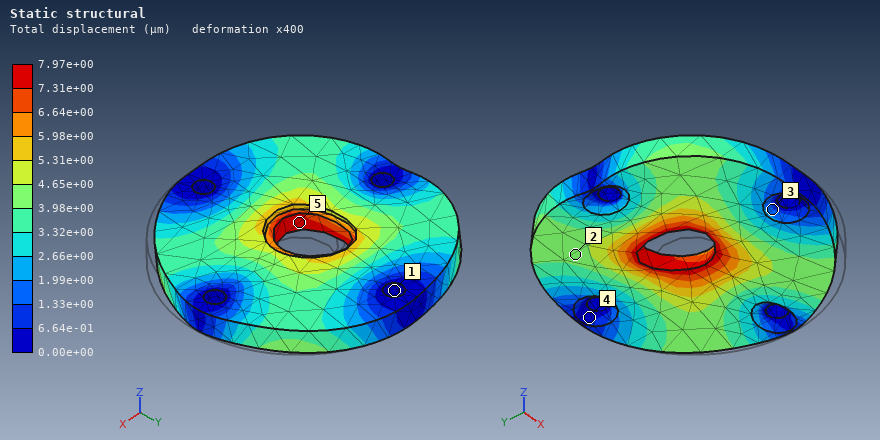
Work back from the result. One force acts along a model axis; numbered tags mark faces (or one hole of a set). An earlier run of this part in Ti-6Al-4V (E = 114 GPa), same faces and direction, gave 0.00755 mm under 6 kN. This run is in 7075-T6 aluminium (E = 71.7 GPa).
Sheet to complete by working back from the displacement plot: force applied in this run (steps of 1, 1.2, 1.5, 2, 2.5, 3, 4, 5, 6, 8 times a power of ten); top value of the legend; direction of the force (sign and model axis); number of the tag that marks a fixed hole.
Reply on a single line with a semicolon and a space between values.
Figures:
4 kN; 7.97e+00 µm; -X; 1
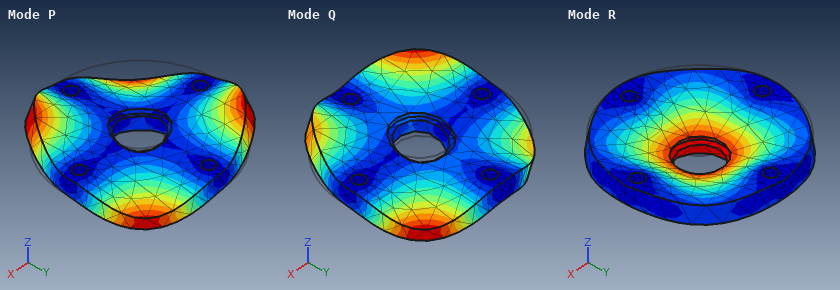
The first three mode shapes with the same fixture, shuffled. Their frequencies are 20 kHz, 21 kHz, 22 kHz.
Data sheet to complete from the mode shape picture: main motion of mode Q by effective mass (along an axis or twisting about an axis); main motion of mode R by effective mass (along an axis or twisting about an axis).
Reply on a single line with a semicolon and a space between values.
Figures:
twisting about X; along Z
